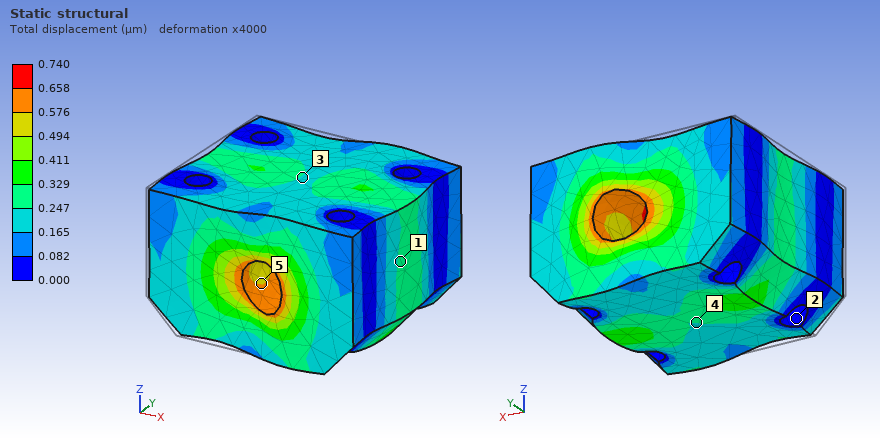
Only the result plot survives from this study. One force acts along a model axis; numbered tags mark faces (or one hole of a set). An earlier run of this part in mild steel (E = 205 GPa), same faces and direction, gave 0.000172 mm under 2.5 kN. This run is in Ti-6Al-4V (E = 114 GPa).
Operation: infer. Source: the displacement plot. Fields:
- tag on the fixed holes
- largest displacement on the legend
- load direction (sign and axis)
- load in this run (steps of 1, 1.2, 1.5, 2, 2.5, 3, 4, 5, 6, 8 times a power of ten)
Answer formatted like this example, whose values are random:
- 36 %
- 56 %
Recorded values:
- 2
- 0.740 µm
- +X
- 6 kN
